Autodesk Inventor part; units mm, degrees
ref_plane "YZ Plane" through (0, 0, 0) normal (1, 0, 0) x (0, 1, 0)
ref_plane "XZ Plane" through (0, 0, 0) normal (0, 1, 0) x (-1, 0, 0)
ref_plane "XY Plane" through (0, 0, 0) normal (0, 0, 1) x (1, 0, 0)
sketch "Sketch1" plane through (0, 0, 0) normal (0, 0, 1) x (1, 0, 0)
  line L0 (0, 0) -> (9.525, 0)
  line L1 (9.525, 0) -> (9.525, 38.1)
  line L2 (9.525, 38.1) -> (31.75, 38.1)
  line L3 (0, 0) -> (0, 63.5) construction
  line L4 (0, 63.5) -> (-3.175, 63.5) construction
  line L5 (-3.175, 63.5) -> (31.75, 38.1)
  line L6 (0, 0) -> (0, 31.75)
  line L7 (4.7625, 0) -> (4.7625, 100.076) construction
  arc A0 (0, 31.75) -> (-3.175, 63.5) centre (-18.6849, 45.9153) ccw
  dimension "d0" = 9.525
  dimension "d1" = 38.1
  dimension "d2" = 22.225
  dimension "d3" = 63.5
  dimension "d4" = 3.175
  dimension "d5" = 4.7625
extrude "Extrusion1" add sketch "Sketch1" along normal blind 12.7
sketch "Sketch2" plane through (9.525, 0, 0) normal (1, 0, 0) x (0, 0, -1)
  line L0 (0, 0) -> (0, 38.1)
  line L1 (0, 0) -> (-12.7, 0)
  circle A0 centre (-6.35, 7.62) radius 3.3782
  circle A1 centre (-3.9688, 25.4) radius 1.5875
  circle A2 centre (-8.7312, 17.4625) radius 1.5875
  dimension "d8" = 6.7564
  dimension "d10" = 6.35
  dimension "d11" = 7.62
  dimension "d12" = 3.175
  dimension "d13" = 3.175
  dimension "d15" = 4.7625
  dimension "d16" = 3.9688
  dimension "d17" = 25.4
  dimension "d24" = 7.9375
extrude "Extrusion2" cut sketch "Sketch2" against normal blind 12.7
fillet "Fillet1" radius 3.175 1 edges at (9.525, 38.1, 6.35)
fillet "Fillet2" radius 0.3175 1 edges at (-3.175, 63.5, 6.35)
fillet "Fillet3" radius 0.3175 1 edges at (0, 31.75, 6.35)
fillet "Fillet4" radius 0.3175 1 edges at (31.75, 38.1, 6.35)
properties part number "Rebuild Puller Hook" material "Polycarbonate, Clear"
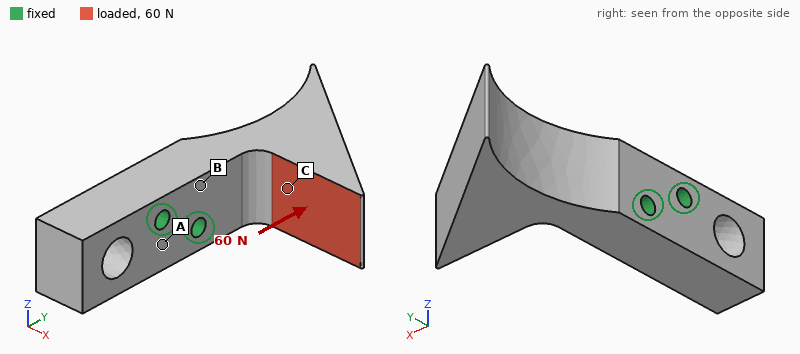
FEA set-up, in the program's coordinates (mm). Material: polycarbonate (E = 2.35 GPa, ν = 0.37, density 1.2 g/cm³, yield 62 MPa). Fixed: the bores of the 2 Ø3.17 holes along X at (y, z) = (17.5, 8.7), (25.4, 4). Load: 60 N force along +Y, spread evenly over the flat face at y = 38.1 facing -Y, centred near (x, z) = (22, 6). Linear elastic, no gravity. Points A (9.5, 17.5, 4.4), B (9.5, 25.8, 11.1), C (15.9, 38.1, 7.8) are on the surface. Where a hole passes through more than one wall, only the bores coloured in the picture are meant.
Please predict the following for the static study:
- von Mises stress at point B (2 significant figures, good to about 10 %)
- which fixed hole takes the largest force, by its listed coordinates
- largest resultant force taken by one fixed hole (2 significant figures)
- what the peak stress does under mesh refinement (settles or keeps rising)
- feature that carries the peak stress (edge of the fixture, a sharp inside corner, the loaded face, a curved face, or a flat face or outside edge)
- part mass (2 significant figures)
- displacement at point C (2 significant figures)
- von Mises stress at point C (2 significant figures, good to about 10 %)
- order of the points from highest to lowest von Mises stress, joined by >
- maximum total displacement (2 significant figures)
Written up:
3.6 MPa
(25.4, 4)
48 N
keeps rising
edge of the fixture
9.2 g
0.14 mm
1.8 MPa
B > C > A
0.38 mm
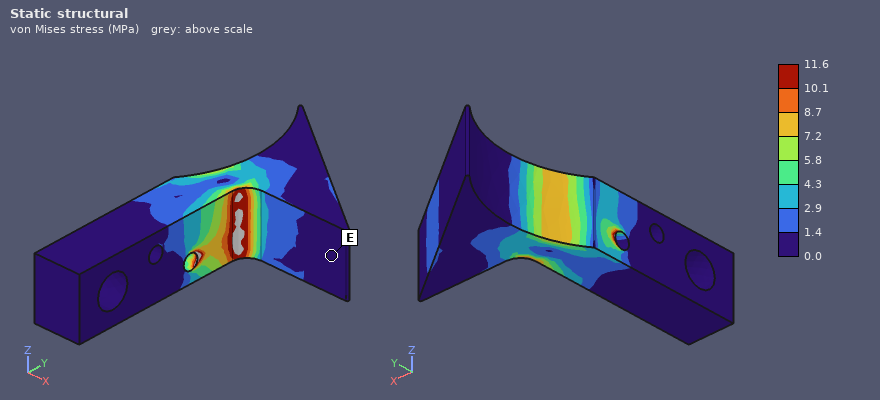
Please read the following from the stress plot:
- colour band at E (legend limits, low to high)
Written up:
0.0 to 1.4 MPa
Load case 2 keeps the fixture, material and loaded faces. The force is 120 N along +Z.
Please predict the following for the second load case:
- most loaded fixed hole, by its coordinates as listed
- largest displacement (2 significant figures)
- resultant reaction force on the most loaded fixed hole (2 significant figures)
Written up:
(25.4, 4)
0.73 mm
210 N
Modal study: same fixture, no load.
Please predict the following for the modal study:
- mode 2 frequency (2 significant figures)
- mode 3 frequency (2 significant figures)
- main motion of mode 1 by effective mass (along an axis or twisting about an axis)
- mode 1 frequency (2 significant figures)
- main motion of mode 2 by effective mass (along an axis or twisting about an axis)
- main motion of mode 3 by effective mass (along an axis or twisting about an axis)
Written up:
1700 Hz
2400 Hz
along X
1300 Hz
along Z
twisting about Y
